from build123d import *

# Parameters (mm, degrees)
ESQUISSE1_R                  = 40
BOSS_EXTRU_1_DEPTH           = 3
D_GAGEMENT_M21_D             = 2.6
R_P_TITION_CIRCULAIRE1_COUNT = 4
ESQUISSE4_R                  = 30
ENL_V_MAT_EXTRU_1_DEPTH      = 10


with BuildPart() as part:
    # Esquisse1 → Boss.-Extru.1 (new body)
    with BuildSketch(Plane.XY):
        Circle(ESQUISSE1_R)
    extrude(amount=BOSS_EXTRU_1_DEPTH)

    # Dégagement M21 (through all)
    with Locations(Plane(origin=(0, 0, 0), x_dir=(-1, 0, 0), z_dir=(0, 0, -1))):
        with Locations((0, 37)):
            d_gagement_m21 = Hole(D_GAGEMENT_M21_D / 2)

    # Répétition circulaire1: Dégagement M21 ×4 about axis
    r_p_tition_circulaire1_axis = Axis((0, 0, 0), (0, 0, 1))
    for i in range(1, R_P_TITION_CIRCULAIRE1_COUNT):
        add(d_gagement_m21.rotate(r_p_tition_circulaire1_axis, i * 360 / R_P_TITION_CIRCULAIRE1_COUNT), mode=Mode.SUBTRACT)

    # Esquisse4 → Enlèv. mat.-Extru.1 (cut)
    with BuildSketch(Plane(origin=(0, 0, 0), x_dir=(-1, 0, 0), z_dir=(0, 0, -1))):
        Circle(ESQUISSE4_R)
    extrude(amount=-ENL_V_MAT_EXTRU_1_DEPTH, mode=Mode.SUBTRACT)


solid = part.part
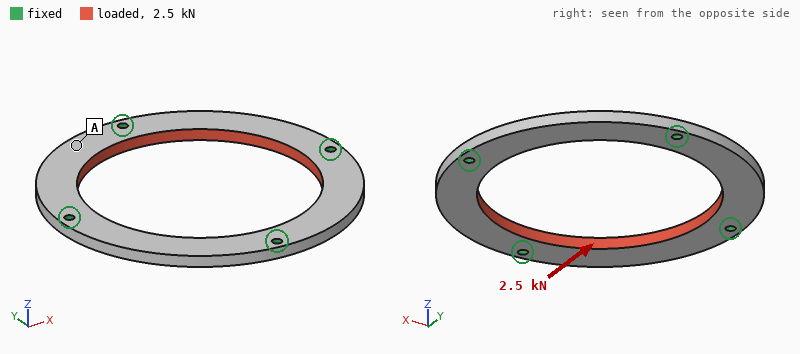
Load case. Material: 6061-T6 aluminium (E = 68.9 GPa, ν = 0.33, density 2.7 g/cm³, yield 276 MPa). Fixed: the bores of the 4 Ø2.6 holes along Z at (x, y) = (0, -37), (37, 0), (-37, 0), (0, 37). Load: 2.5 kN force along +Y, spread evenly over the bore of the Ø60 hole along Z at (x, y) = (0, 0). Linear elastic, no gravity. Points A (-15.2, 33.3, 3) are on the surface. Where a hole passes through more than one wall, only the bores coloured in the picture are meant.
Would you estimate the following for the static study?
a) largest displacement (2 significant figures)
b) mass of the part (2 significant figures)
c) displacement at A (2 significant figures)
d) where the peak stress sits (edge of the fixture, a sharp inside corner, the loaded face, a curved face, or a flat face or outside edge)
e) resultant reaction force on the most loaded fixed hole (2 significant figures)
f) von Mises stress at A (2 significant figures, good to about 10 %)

9.8 µm
18 g
7.1 µm
edge of the fixture
890 N
8.8 MPa
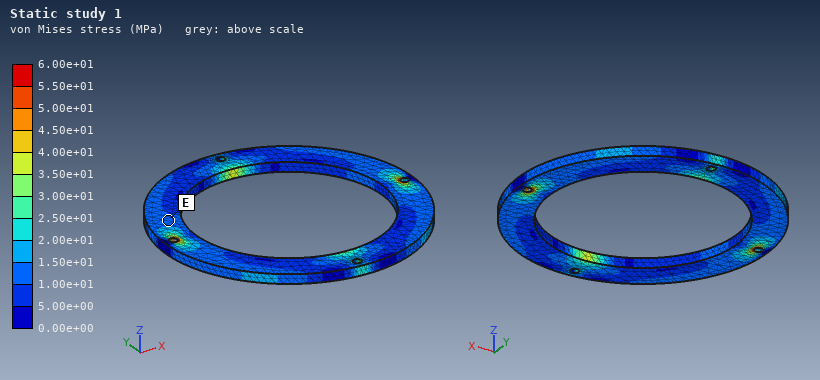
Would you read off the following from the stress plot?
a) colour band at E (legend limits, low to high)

1.00e+01 to 1.50e+01 MPa
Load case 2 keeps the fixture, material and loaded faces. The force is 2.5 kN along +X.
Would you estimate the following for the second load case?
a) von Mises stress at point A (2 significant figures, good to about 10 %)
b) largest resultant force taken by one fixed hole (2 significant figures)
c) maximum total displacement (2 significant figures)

12 MPa
890 N
9.8 µm
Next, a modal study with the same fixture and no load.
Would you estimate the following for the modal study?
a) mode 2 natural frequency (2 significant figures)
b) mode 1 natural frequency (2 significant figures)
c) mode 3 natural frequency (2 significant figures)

4600 Hz
4400 Hz
4600 Hz
